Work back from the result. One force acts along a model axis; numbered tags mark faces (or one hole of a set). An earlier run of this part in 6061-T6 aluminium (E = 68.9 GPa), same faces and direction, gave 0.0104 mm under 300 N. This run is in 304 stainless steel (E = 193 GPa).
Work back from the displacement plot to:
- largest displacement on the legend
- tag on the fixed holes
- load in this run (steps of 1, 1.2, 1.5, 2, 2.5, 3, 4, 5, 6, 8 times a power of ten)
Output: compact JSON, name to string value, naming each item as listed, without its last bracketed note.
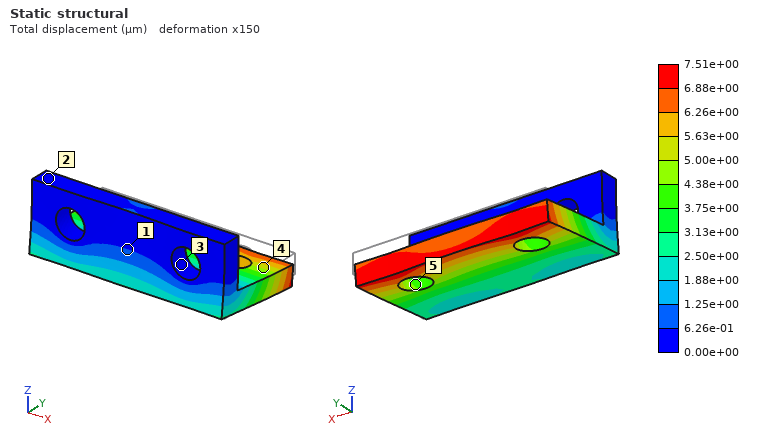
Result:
{"largest displacement on the legend": "7.51e+00 µm", "tag on the fixed holes": "3", "load in this run": "600 N"}
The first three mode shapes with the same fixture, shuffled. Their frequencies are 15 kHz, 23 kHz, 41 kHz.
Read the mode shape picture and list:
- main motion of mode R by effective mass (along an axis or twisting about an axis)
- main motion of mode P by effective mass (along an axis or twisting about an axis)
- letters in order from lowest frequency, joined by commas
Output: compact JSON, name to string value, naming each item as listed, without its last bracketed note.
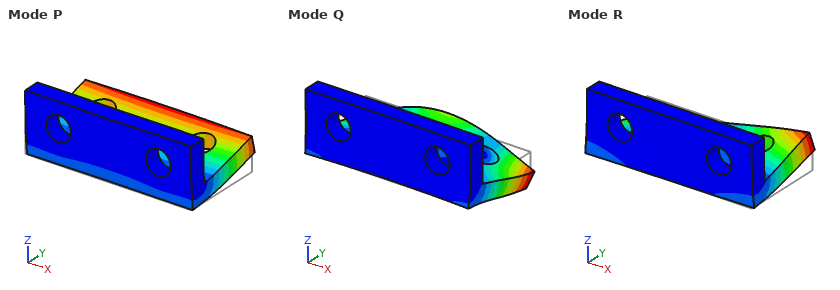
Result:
{"main motion of mode R by effective mass": "twisting about Y", "main motion of mode P by effective mass": "along Z", "letters in order from lowest frequency, joined by commas": "P, R, Q"}
